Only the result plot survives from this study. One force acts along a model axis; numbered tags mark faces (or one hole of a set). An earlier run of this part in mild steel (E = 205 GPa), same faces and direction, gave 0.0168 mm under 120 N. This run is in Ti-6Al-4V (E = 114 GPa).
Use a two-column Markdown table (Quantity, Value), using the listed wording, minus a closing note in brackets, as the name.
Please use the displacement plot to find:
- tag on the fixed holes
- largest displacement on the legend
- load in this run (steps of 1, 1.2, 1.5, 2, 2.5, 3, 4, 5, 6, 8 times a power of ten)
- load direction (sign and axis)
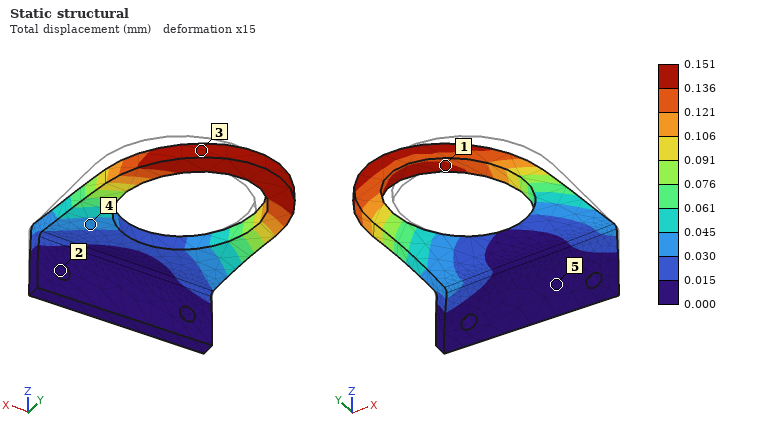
| Quantity | Value |
|---|---|
| tag on the fixed holes | 2 |
| largest displacement on the legend | 0.151 mm |
| load in this run | 600 N |
| load direction | -X |
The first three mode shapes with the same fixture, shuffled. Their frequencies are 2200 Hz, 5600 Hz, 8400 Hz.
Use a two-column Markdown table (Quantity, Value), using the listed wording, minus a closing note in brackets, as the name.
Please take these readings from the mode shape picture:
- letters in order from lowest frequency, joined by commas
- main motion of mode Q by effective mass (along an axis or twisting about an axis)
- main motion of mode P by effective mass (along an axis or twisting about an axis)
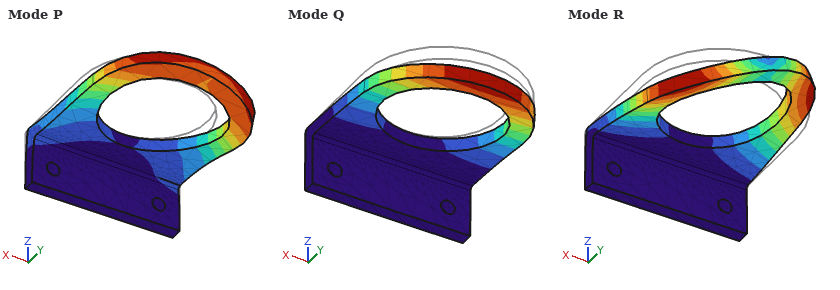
| Quantity | Value |
|---|---|
| letters in order from lowest frequency, joined by commas | Q, R, P |
| main motion of mode Q by effective mass | along Z |
| main motion of mode P by effective mass | along X |
